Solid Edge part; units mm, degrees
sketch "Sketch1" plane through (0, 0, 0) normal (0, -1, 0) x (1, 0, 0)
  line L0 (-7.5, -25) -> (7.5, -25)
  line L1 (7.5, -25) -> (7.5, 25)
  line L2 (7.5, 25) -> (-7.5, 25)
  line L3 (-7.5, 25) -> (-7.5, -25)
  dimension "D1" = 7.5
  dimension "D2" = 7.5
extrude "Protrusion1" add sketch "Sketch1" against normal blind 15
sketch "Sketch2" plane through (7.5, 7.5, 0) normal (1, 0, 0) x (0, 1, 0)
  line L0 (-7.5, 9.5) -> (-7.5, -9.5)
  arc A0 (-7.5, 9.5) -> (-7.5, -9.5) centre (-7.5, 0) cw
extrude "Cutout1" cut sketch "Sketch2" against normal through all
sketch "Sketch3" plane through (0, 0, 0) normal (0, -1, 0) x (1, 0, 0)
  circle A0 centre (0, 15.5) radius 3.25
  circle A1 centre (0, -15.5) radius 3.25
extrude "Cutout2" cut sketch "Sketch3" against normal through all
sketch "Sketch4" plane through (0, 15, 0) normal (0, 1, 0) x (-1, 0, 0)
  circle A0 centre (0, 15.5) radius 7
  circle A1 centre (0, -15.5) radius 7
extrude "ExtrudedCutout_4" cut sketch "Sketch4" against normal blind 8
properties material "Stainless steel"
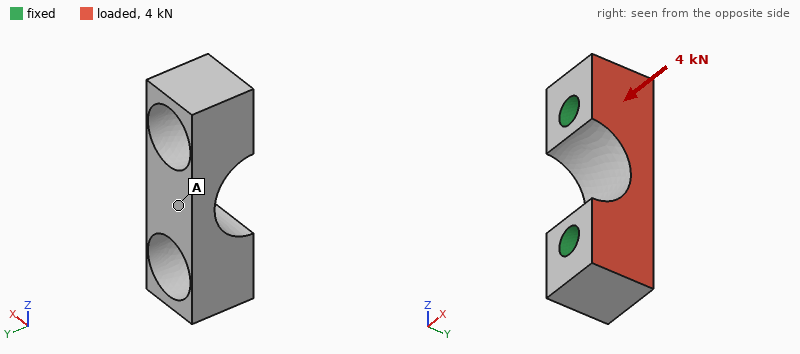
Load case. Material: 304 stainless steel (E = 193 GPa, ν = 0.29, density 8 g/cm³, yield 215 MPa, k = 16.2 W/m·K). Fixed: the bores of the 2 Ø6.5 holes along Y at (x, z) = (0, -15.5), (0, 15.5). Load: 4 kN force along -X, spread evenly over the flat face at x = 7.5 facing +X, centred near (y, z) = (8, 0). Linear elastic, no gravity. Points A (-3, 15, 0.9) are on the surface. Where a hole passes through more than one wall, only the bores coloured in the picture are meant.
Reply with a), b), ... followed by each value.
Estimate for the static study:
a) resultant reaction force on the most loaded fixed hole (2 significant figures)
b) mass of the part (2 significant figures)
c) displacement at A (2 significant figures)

a) 2.0 kN
b) 50 g
c) 5.2 µm
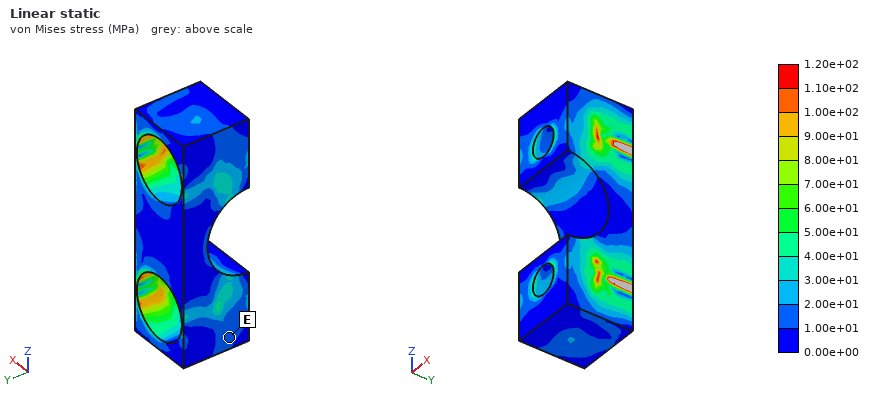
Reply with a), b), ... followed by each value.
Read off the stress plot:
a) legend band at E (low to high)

a) 1.00e+01 to 2.00e+01 MPa
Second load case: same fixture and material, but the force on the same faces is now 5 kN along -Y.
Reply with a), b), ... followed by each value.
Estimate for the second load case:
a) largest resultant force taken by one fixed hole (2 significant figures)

a) 2.5 kN
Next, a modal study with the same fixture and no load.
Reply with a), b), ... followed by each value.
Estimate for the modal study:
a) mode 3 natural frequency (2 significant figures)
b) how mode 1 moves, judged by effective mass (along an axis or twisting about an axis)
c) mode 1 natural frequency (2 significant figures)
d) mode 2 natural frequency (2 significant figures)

a) 30 kHz
b) along X
c) 21 kHz
d) 30 kHz
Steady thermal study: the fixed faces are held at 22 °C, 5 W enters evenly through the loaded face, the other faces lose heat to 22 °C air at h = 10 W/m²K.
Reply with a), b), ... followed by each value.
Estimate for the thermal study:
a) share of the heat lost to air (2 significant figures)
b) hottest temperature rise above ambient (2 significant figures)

a) 3.1 %
b) 16 K
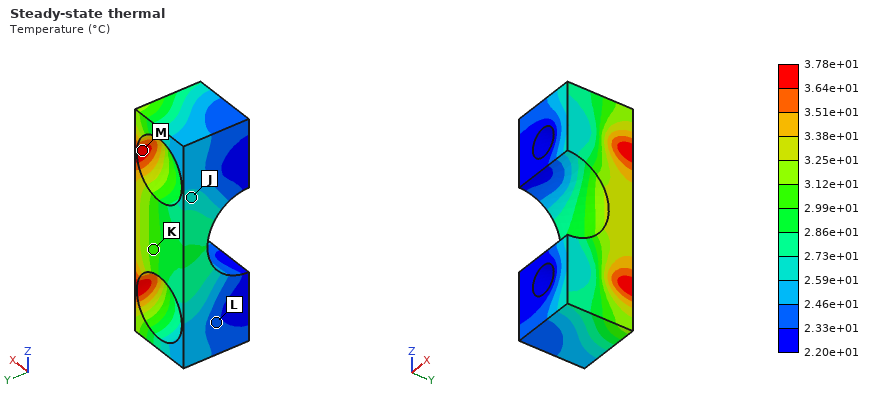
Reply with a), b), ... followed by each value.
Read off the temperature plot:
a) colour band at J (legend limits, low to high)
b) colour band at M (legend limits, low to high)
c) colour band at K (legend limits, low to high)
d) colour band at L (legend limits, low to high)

a) 2.59e+01 to 2.73e+01 °C
b) 3.64e+01 to 3.78e+01 °C
c) 2.99e+01 to 3.12e+01 °C
d) 2.33e+01 to 2.46e+01 °C
